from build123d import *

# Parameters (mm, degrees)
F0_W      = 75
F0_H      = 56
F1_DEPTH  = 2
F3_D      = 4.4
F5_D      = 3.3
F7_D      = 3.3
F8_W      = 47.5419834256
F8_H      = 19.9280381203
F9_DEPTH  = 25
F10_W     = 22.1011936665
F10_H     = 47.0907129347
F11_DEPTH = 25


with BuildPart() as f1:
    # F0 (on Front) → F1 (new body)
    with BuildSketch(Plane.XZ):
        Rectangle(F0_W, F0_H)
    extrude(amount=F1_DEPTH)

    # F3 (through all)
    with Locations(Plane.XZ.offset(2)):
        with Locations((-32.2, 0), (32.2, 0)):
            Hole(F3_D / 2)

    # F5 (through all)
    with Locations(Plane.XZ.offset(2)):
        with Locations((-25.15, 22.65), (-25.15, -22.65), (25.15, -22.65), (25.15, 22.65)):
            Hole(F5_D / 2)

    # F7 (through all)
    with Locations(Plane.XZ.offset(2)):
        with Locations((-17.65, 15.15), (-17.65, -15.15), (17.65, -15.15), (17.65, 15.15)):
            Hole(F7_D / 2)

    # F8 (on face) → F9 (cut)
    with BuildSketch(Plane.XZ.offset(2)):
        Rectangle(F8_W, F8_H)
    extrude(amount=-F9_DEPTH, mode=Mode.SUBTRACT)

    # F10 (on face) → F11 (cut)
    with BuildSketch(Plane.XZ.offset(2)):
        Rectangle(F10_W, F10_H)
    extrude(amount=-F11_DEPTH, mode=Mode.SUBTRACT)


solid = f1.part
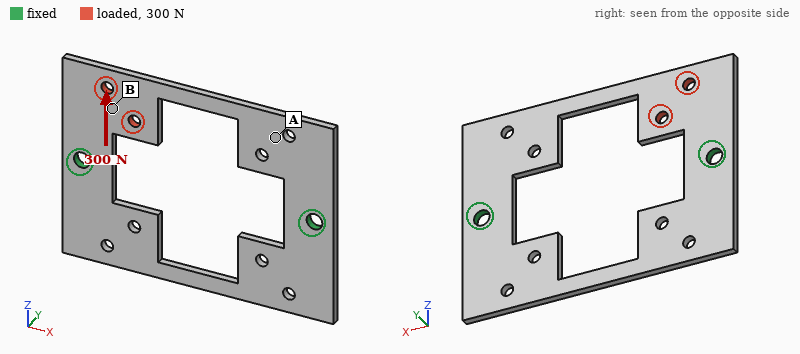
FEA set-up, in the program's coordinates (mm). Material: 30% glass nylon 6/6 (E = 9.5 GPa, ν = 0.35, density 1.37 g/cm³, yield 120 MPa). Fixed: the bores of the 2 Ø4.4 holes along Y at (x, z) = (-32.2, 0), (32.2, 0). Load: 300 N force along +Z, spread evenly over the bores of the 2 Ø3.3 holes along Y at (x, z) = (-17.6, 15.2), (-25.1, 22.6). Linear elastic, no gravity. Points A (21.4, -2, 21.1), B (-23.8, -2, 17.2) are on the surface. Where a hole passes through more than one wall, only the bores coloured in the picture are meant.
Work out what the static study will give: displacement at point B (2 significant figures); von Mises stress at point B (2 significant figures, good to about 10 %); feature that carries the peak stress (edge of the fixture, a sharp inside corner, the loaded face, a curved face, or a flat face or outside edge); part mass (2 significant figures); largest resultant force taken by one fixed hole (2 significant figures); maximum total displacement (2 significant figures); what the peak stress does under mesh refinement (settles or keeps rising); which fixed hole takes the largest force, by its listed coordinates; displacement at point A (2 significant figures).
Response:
0.085 mm
15 MPa
edge of the fixture
7.0 g
280 N
0.15 mm
keeps rising
(-32.2, 0)
0.069 mm
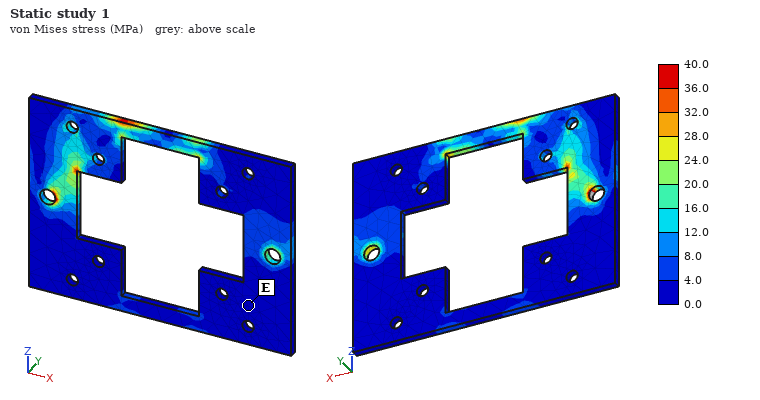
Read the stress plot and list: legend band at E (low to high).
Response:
0.0 to 4.0 MPa
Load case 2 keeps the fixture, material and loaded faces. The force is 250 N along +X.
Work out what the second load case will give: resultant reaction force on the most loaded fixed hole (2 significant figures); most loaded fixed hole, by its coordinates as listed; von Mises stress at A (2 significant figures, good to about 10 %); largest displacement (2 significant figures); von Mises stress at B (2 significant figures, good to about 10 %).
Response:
180 N
(-32.2, 0)
4.3 MPa
0.18 mm
5.8 MPa
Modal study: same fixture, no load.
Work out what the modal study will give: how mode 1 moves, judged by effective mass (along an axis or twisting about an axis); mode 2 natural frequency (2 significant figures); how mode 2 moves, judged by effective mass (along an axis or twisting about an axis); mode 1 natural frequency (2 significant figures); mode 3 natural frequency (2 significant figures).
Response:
twisting about X
720 Hz
along Y
690 Hz
1200 Hz
